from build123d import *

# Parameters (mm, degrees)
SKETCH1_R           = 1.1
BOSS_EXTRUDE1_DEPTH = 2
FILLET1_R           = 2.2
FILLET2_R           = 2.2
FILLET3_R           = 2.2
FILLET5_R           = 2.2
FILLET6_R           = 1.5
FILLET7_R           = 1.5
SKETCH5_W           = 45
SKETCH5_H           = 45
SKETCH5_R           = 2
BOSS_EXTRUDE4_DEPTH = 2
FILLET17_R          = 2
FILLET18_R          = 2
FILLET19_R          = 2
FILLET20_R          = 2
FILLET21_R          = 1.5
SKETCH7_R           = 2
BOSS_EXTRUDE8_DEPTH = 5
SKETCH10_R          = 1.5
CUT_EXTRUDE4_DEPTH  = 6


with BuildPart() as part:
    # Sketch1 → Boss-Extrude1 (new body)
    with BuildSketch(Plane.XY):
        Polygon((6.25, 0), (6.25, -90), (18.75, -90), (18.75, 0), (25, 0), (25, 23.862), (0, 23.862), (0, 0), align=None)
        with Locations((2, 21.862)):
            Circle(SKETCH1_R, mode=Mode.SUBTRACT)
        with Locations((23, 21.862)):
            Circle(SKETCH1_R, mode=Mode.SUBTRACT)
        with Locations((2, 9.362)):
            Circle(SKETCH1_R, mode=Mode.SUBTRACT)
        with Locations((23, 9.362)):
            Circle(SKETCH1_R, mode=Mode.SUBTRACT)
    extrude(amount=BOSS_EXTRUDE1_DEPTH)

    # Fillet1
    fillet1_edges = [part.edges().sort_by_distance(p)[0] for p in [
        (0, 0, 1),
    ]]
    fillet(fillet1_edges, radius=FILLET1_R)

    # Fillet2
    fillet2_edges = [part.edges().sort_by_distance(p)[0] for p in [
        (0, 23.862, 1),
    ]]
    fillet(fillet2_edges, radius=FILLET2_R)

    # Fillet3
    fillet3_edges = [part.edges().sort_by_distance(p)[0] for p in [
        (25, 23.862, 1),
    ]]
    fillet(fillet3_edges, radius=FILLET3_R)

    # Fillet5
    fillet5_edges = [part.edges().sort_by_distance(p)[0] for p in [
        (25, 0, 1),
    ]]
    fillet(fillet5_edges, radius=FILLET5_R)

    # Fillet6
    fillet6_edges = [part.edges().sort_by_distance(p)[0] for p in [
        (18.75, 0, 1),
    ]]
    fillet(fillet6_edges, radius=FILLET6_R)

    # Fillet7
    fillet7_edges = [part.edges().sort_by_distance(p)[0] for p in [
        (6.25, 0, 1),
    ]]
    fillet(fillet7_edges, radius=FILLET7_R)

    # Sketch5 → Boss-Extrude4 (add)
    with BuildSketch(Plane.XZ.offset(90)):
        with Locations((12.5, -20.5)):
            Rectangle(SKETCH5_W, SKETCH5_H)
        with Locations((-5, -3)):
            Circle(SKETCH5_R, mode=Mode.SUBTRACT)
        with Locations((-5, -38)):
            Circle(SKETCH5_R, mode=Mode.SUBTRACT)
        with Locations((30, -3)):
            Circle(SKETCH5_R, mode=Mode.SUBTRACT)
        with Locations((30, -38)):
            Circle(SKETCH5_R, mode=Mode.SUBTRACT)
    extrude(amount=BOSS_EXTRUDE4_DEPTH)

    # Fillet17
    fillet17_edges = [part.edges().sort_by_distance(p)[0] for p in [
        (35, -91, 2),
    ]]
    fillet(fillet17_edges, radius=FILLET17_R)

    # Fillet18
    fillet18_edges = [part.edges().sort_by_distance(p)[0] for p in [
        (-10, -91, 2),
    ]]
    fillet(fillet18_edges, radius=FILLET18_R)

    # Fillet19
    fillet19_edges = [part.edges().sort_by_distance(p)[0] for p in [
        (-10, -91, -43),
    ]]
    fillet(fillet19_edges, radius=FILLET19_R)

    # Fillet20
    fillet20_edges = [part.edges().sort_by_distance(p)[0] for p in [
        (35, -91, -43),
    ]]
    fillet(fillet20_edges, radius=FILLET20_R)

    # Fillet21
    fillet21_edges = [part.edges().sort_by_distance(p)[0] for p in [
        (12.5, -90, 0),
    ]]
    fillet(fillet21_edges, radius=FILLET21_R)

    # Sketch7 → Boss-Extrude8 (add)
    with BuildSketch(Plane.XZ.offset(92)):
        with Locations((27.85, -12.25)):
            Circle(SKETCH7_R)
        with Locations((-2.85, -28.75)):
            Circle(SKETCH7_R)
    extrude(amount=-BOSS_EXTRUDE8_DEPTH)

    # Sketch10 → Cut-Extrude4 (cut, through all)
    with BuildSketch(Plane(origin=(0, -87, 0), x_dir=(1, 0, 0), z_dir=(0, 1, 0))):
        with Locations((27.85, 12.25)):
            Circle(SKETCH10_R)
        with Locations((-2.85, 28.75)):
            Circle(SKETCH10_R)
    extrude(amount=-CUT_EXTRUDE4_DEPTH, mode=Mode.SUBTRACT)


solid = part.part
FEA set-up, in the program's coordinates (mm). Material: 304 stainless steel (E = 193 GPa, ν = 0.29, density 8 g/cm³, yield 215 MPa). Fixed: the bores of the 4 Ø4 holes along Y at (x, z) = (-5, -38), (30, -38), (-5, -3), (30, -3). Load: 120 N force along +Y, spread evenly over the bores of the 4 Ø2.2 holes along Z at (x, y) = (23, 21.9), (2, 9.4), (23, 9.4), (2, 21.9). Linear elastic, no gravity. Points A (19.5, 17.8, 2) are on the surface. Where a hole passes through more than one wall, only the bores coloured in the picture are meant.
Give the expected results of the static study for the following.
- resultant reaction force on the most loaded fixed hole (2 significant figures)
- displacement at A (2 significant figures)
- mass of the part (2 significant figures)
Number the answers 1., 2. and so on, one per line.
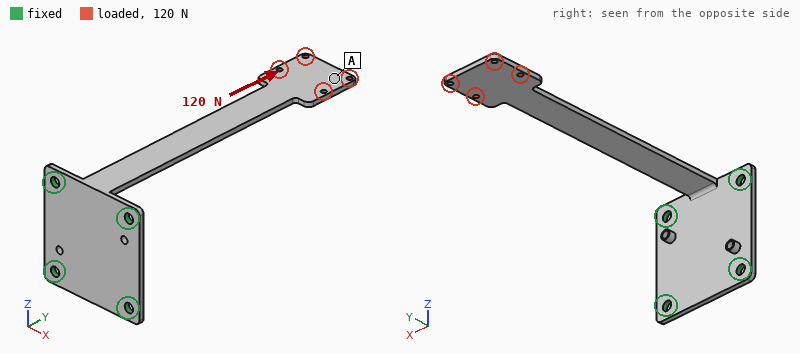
1. 68 N
2. 0.11 mm
3. 59 g
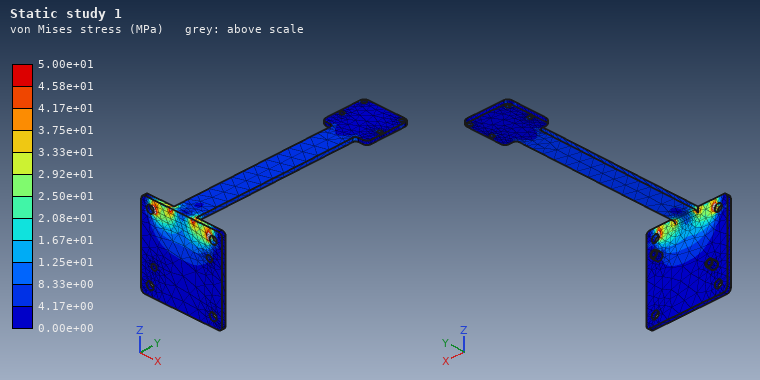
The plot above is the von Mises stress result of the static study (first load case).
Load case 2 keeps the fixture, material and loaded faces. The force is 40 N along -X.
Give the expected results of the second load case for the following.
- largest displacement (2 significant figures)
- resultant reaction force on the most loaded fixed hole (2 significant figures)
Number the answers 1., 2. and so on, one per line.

1. 0.62 mm
2. 190 N
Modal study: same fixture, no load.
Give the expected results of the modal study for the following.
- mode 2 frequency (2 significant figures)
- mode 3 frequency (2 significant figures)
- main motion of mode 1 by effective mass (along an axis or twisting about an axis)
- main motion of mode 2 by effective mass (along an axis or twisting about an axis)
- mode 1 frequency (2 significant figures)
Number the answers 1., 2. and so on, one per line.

1. 390 Hz
2. 670 Hz
3. along Z
4. along X
5. 92 Hz
